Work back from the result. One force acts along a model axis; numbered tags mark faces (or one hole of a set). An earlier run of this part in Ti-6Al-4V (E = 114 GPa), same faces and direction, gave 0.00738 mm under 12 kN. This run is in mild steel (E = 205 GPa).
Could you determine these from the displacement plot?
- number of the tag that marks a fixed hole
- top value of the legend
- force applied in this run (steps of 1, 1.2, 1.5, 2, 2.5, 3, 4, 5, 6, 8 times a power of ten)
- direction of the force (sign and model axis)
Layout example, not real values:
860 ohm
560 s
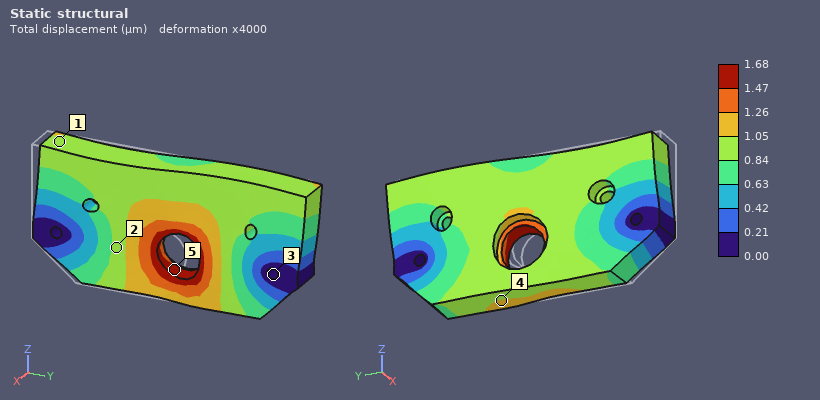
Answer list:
3
1.68 µm
5 kN
+Y
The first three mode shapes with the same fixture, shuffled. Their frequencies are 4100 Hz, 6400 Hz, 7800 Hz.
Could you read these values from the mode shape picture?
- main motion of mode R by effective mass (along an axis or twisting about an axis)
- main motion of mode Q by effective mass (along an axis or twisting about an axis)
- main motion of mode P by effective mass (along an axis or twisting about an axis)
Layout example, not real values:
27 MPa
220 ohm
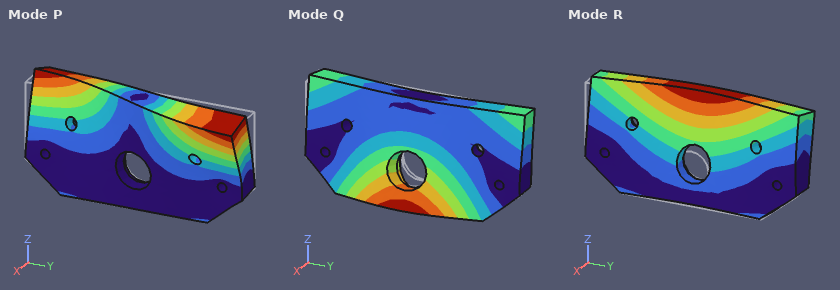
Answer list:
along X
along X
twisting about Z
